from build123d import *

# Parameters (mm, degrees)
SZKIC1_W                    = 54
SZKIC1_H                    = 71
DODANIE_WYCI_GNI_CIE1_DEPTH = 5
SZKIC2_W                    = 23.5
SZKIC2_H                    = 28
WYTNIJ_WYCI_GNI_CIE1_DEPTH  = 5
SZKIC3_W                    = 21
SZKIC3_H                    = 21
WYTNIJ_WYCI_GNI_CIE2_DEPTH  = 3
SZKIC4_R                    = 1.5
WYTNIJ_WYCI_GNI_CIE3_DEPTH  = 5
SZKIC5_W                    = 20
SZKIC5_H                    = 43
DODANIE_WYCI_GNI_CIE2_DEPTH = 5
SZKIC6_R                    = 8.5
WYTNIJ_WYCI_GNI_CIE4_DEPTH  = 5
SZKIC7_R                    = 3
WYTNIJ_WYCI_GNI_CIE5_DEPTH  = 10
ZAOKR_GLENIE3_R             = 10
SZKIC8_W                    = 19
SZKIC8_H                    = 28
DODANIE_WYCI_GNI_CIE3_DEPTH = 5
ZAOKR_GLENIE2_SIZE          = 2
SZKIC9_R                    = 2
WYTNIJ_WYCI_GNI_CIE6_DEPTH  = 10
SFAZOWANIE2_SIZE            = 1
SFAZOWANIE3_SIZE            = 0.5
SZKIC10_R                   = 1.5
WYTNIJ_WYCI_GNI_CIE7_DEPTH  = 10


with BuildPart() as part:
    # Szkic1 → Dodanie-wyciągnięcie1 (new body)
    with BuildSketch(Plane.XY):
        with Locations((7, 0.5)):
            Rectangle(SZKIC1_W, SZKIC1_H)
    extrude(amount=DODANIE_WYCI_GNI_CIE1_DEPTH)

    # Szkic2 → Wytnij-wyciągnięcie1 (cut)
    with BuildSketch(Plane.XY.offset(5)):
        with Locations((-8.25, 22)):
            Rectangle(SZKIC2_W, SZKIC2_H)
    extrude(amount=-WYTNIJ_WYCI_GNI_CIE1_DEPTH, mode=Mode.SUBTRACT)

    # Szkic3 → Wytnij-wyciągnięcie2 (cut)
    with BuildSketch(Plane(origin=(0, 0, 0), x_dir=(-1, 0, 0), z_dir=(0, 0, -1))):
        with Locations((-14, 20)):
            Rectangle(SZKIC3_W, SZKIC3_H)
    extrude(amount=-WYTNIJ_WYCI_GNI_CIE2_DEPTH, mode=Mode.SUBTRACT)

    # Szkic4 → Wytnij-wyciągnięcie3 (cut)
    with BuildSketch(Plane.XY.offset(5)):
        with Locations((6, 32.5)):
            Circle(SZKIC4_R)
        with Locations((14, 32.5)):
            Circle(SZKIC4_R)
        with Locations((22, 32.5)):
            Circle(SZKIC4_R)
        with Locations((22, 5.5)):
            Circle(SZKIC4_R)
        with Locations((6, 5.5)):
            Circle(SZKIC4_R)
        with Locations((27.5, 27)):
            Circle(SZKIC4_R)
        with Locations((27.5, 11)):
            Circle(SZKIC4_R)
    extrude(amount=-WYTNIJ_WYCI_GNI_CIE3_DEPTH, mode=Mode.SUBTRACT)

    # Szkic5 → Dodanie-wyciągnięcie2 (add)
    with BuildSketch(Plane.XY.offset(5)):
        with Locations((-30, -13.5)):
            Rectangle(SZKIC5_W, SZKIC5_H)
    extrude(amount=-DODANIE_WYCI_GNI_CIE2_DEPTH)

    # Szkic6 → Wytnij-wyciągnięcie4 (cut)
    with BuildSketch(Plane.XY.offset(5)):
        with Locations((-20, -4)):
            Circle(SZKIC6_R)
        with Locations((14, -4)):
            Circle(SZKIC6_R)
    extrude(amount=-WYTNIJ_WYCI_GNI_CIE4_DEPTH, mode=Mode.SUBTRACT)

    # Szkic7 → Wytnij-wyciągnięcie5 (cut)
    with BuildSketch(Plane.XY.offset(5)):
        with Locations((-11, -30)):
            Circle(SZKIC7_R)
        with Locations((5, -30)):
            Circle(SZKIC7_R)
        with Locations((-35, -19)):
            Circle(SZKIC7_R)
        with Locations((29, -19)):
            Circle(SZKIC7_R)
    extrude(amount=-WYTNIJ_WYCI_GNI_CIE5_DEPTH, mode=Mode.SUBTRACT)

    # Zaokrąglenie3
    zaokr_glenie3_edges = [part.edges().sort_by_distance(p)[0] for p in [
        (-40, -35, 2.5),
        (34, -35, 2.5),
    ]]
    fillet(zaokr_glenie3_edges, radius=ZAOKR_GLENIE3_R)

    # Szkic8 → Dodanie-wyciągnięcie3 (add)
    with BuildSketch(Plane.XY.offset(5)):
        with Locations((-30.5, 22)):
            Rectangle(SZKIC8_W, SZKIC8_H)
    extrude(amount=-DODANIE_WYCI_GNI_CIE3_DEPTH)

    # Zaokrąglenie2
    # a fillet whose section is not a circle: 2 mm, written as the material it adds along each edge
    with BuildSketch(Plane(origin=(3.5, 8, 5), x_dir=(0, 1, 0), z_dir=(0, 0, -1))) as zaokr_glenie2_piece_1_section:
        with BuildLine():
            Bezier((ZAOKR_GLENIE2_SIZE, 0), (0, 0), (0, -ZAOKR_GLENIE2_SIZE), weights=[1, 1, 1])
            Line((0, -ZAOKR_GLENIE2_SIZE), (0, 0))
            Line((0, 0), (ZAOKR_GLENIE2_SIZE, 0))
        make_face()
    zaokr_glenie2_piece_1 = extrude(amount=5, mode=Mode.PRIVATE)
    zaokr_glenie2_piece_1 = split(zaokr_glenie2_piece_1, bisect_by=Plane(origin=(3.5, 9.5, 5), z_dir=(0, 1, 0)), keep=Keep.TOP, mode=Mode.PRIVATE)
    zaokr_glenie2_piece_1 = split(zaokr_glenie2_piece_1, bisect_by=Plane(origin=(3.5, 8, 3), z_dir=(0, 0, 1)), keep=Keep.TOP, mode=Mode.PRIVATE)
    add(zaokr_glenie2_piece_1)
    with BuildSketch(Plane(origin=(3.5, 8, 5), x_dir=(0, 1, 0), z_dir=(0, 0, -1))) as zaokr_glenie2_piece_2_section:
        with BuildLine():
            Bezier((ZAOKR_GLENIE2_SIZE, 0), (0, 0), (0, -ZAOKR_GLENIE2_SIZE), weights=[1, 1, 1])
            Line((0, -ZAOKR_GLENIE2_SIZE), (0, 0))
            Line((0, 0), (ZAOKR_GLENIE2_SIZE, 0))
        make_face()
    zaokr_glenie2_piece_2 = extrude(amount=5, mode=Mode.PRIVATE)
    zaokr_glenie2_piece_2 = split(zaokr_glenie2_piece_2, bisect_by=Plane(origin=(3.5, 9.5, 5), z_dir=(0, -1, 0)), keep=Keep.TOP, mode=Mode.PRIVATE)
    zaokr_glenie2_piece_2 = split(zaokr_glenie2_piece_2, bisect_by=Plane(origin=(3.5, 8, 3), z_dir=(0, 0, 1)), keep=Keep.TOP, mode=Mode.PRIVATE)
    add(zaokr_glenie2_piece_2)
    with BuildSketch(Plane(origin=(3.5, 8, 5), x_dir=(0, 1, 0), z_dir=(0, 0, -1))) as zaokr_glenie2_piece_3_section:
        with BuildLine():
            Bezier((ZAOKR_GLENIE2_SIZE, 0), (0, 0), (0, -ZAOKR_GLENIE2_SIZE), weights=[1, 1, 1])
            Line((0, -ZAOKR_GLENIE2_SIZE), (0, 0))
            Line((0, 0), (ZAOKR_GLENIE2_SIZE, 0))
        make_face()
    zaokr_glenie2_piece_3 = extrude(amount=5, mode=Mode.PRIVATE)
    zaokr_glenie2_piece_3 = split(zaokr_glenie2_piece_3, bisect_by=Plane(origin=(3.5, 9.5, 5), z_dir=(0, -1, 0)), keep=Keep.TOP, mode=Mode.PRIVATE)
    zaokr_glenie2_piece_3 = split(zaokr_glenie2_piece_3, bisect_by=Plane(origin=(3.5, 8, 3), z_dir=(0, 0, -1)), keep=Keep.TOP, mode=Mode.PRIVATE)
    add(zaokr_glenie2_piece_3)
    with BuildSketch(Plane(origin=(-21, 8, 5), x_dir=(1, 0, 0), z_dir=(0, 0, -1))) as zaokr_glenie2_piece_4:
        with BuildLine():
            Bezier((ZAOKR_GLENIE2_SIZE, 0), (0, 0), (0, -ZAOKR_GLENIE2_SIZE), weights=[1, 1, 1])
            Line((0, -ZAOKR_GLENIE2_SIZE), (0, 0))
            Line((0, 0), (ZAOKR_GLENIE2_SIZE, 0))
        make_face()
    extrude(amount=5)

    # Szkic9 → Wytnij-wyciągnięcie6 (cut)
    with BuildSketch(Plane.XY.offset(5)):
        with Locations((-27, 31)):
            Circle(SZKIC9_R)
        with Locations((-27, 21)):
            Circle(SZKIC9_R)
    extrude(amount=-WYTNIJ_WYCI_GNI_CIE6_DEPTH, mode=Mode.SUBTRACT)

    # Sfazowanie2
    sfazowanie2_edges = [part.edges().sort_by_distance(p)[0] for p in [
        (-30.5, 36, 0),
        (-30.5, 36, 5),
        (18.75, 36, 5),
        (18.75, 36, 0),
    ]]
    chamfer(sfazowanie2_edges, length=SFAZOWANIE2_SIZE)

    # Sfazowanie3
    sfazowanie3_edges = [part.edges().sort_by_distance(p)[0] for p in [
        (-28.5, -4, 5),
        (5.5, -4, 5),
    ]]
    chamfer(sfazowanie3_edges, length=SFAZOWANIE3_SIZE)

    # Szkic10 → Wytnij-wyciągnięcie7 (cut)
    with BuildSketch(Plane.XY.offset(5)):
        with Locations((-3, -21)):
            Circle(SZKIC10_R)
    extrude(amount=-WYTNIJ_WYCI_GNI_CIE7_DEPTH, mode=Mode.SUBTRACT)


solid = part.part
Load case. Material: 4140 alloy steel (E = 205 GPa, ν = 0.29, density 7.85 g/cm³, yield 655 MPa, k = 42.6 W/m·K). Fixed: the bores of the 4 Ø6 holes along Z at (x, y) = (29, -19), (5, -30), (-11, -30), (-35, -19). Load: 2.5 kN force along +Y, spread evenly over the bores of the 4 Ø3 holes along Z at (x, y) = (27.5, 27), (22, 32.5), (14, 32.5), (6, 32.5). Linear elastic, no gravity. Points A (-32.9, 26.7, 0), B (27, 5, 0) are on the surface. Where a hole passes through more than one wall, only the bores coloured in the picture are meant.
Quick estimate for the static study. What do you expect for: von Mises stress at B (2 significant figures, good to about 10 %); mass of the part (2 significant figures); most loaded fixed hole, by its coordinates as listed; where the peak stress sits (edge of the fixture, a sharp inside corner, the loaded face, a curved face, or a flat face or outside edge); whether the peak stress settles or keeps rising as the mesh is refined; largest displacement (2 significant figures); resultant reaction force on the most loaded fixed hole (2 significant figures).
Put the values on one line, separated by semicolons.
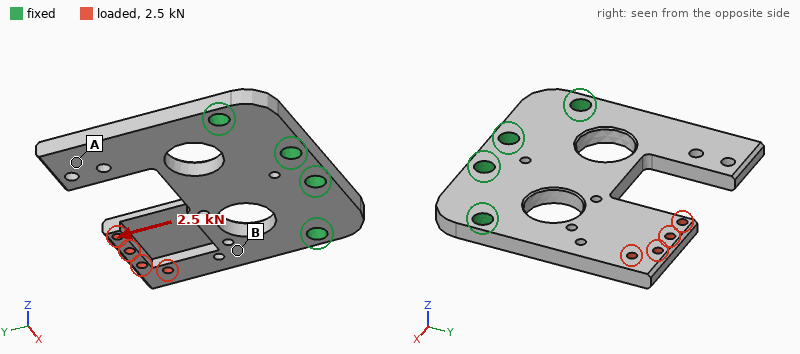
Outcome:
46 MPa; 140 g; (29, -19); a sharp inside corner; keeps rising; 80 µm; 1.6 kN
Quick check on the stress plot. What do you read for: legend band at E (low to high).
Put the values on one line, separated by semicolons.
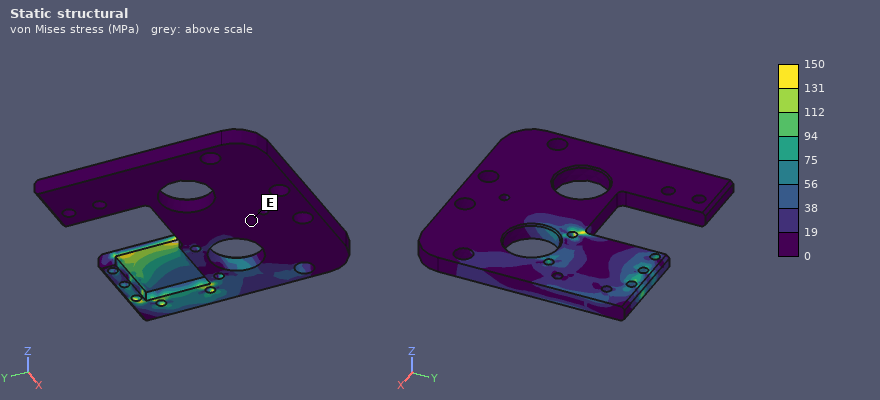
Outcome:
0 to 19 MPa
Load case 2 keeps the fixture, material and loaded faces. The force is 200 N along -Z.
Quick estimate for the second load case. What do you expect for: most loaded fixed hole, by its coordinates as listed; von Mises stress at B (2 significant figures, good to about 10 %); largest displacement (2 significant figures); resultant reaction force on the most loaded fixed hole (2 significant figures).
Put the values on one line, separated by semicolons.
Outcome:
(29, -19); 71 MPa; 0.24 mm; 190 N
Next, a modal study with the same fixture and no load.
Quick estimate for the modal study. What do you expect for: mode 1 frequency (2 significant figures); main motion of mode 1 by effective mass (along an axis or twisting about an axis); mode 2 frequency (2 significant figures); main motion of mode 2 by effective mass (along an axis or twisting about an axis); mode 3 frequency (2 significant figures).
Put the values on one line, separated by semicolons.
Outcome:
1400 Hz; along Z; 1600 Hz; twisting about Y; 4300 Hz
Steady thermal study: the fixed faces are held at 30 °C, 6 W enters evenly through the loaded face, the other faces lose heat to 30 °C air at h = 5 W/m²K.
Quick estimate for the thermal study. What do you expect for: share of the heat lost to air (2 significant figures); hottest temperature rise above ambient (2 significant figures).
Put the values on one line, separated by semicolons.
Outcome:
12 %; 74 K
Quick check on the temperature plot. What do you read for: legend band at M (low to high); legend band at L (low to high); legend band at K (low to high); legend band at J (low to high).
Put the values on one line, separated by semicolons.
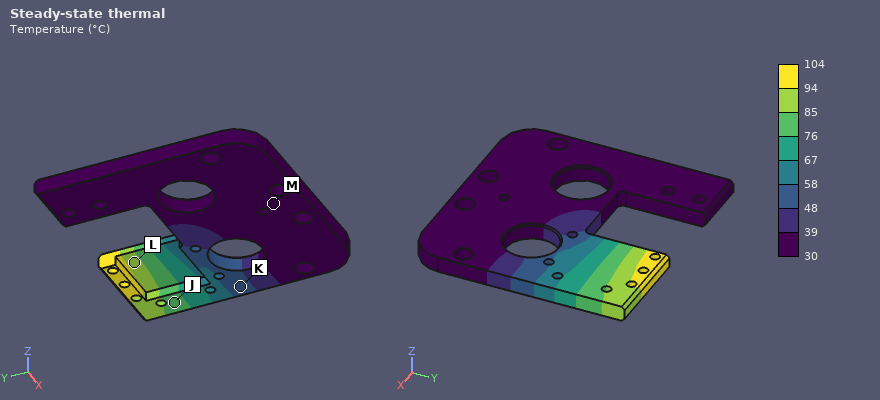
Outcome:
30 to 39 °C; 85 to 94 °C; 48 to 58 °C; 76 to 85 °C
